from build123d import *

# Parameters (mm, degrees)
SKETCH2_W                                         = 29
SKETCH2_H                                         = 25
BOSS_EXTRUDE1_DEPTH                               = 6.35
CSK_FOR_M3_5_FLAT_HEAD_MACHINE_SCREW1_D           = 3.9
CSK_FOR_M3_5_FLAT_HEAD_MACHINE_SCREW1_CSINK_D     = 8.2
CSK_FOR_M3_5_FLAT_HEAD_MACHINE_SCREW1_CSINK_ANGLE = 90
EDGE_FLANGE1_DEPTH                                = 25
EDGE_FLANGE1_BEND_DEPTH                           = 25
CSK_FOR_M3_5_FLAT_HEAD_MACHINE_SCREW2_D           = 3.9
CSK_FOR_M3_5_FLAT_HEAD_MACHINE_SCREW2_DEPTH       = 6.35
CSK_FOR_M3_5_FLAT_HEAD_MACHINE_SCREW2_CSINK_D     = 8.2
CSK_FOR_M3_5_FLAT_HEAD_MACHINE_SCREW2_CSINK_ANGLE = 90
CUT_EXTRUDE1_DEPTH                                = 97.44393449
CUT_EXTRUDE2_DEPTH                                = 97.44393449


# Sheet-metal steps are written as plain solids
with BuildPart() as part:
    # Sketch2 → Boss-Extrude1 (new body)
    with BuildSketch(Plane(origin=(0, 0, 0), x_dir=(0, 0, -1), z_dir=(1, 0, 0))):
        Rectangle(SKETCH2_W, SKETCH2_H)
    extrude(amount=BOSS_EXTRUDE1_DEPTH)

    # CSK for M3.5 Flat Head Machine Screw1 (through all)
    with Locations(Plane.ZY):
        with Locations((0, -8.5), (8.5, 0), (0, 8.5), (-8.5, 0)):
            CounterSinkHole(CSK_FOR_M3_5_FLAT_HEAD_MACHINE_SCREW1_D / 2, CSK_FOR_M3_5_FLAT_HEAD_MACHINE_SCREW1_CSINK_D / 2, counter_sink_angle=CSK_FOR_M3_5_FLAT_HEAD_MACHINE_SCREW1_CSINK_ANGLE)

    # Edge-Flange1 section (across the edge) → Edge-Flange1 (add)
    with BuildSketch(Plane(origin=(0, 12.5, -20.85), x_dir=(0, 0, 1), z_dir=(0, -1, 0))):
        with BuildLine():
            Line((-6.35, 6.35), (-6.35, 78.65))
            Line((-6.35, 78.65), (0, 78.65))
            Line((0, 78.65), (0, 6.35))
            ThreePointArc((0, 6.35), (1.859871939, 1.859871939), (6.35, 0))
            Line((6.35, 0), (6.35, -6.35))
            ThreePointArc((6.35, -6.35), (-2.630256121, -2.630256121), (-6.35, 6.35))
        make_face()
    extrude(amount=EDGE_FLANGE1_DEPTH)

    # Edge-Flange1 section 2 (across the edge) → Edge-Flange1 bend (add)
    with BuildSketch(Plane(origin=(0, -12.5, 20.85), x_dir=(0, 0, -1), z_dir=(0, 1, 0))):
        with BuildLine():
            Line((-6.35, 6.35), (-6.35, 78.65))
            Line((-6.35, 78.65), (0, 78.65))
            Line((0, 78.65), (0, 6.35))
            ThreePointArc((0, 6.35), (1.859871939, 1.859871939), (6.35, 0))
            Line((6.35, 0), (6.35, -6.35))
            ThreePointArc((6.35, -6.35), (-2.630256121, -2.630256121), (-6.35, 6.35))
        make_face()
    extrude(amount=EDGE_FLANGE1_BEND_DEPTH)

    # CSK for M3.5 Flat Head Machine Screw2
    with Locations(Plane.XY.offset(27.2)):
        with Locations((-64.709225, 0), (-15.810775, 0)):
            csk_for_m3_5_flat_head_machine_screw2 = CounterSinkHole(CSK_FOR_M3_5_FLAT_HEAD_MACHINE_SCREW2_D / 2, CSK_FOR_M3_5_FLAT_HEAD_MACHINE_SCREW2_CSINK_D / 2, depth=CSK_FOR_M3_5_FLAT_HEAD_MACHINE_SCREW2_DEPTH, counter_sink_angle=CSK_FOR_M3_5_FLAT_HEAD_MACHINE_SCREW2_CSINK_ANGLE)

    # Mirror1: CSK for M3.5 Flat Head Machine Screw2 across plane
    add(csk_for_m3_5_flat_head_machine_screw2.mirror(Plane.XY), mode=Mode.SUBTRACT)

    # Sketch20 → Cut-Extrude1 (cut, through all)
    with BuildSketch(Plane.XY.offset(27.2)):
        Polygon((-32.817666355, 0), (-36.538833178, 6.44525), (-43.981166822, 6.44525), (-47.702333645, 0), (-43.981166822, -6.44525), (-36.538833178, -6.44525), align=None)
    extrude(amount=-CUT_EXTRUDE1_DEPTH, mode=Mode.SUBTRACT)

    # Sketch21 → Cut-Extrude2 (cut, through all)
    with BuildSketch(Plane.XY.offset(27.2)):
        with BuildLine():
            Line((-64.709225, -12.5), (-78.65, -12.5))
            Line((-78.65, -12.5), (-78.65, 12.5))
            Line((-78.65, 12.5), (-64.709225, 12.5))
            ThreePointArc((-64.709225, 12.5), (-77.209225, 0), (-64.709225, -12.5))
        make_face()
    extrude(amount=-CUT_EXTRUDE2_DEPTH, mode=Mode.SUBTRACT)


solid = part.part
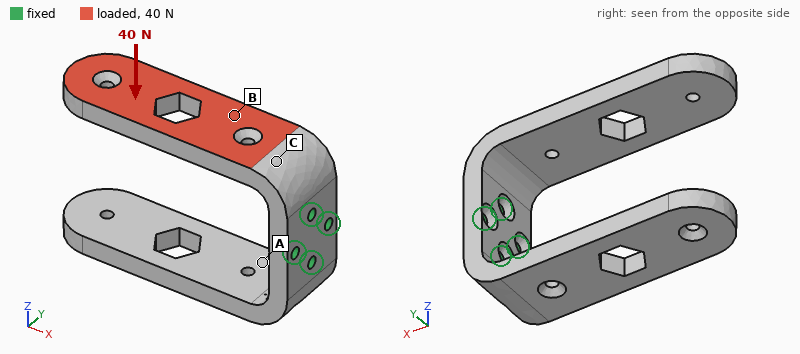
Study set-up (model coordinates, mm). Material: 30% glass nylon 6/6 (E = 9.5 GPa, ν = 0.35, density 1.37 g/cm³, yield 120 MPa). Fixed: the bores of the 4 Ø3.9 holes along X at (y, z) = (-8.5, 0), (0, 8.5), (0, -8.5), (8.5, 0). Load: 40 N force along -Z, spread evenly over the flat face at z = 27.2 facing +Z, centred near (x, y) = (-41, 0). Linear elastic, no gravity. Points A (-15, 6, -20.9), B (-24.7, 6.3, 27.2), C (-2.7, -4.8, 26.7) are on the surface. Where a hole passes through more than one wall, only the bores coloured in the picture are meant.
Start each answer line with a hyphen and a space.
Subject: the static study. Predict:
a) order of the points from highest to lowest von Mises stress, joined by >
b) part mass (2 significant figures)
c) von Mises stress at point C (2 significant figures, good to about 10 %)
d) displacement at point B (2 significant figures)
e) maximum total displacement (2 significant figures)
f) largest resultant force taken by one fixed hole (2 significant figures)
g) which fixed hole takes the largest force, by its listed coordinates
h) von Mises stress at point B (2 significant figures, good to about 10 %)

- C > B > A
- 39 g
- 6.6 MPa
- 0.26 mm
- 1.00 mm
- 120 N
- (0, 8.5)
- 4.5 MPa
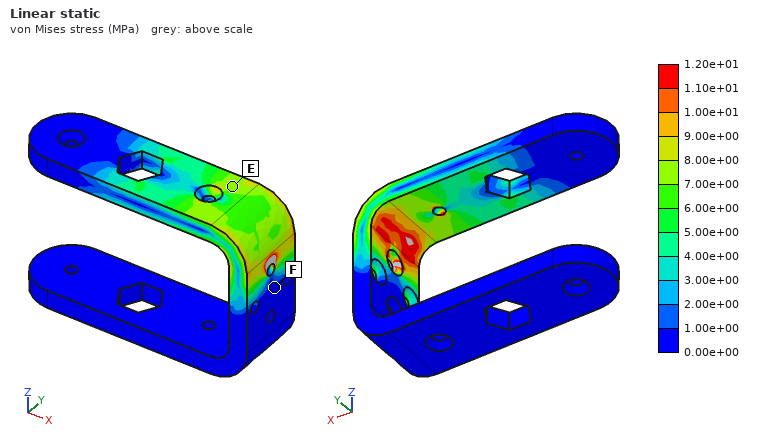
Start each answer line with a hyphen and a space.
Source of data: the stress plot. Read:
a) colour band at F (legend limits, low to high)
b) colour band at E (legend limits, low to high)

- 0.00e+00 to 1.00e+00 MPa
- 7.00e+00 to 8.00e+00 MPa
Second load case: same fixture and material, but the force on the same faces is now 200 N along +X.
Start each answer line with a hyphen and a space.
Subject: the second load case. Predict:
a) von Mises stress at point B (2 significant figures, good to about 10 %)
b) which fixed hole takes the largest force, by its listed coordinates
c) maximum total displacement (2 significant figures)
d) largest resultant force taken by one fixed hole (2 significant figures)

- 3.7 MPa
- (0, 8.5)
- 1.0 mm
- 390 N
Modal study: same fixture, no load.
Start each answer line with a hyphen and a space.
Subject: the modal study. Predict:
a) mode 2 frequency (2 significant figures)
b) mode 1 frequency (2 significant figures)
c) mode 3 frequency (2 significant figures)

- 350 Hz
- 340 Hz
- 570 Hz
